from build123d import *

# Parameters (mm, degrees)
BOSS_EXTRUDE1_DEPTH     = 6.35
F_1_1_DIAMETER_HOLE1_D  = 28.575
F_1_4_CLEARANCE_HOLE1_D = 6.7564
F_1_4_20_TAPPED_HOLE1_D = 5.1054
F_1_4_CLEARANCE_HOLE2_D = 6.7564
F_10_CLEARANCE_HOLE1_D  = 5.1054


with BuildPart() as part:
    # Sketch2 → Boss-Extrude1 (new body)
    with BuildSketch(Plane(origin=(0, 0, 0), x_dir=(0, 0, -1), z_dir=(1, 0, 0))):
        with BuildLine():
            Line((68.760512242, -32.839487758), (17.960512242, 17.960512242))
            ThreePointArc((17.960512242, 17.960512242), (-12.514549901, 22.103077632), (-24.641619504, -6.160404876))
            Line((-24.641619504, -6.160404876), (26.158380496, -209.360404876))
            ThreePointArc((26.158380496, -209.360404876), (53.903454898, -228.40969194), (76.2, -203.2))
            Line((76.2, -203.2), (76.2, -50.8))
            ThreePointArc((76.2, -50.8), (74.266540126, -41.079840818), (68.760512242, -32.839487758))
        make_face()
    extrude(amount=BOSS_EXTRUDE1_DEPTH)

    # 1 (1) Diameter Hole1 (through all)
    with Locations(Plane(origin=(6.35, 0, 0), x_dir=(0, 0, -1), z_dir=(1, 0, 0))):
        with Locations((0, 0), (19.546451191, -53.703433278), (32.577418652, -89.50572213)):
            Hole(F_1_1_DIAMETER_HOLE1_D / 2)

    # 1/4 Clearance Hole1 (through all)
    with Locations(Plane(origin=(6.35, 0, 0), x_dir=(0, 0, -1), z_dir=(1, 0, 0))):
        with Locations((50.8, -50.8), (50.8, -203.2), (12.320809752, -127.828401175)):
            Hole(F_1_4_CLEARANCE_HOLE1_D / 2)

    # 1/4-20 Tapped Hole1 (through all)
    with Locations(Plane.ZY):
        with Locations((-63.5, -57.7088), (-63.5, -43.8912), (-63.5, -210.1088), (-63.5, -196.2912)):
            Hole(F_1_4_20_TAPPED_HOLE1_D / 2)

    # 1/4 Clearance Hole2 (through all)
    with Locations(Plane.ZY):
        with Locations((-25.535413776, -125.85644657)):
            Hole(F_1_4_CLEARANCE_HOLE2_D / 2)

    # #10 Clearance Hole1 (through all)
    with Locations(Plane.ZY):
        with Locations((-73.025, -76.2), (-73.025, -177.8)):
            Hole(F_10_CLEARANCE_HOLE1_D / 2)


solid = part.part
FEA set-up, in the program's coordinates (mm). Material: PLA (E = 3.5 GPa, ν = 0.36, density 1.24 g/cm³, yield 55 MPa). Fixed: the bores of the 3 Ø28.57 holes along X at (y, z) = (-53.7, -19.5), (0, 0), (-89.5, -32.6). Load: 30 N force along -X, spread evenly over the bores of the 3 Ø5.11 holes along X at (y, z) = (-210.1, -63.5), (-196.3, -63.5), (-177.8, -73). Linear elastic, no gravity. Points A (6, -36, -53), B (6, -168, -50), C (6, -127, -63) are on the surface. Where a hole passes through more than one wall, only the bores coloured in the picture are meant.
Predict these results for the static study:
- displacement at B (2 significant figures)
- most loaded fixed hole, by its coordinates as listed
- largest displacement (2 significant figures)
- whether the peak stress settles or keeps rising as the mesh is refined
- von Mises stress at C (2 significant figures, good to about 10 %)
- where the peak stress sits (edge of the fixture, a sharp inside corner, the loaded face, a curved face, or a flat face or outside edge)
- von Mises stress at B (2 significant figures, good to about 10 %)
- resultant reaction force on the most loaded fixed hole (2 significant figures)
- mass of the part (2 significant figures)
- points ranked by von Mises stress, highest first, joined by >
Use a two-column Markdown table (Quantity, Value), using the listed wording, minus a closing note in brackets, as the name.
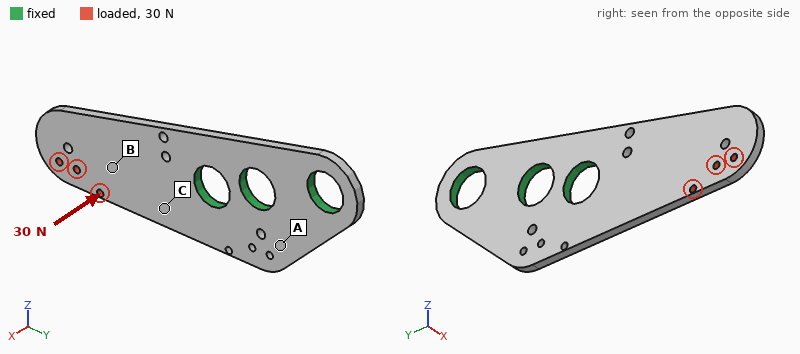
| Quantity | Value |
|---|---|
| displacement at B | 1.1 mm |
| most loaded fixed hole, by its coordinates as listed | (-89.5, -32.6) |
| largest displacement | 2.8 mm |
| whether the peak stress settles or keeps rising as the mesh is refined | keeps rising |
| von Mises stress at C | 4.4 MPa |
| where the peak stress sits | a sharp inside corner |
| von Mises stress at B | 2.3 MPa |
| resultant reaction force on the most loaded fixed hole | 33 N |
| mass of the part | 120 g |
| points ranked by von Mises stress, highest first, joined by > | C > B > A |
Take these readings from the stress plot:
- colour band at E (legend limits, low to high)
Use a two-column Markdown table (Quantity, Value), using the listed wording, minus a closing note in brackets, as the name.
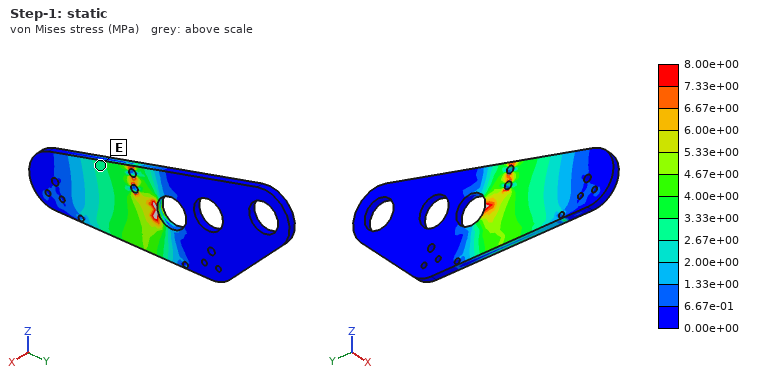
| Quantity | Value |
|---|---|
| colour band at E | 2.67e+00 to 3.33e+00 MPa |
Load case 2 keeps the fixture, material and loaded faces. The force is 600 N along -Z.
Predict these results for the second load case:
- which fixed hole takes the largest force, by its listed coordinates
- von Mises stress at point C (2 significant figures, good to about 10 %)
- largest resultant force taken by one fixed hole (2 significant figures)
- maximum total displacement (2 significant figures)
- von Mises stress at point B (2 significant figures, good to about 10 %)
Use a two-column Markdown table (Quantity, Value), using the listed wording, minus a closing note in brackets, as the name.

| Quantity | Value |
|---|---|
| which fixed hole takes the largest force, by its listed coordinates | (-89.5, -32.6) |
| von Mises stress at point C | 5.0 MPa |
| largest resultant force taken by one fixed hole | 1.0 kN |
| maximum total displacement | 0.84 mm |
| von Mises stress at point B | 3.5 MPa |
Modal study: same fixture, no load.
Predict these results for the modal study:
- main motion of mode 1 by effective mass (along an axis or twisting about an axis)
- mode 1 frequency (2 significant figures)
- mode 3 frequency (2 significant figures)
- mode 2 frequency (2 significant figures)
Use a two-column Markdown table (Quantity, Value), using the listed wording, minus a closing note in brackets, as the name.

| Quantity | Value |
|---|---|
| main motion of mode 1 by effective mass | along X |
| mode 1 frequency | 130 Hz |
| mode 3 frequency | 690 Hz |
| mode 2 frequency | 540 Hz |
